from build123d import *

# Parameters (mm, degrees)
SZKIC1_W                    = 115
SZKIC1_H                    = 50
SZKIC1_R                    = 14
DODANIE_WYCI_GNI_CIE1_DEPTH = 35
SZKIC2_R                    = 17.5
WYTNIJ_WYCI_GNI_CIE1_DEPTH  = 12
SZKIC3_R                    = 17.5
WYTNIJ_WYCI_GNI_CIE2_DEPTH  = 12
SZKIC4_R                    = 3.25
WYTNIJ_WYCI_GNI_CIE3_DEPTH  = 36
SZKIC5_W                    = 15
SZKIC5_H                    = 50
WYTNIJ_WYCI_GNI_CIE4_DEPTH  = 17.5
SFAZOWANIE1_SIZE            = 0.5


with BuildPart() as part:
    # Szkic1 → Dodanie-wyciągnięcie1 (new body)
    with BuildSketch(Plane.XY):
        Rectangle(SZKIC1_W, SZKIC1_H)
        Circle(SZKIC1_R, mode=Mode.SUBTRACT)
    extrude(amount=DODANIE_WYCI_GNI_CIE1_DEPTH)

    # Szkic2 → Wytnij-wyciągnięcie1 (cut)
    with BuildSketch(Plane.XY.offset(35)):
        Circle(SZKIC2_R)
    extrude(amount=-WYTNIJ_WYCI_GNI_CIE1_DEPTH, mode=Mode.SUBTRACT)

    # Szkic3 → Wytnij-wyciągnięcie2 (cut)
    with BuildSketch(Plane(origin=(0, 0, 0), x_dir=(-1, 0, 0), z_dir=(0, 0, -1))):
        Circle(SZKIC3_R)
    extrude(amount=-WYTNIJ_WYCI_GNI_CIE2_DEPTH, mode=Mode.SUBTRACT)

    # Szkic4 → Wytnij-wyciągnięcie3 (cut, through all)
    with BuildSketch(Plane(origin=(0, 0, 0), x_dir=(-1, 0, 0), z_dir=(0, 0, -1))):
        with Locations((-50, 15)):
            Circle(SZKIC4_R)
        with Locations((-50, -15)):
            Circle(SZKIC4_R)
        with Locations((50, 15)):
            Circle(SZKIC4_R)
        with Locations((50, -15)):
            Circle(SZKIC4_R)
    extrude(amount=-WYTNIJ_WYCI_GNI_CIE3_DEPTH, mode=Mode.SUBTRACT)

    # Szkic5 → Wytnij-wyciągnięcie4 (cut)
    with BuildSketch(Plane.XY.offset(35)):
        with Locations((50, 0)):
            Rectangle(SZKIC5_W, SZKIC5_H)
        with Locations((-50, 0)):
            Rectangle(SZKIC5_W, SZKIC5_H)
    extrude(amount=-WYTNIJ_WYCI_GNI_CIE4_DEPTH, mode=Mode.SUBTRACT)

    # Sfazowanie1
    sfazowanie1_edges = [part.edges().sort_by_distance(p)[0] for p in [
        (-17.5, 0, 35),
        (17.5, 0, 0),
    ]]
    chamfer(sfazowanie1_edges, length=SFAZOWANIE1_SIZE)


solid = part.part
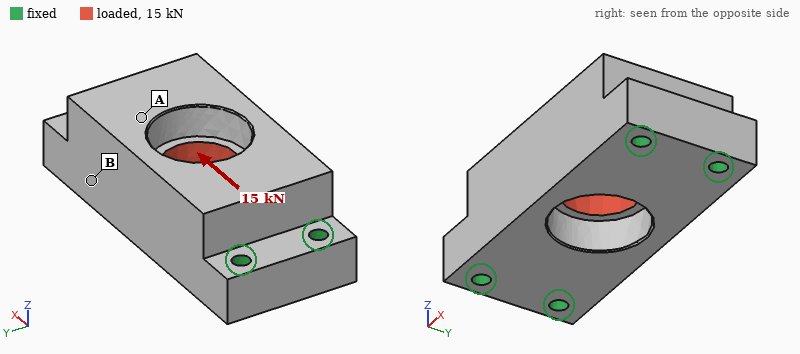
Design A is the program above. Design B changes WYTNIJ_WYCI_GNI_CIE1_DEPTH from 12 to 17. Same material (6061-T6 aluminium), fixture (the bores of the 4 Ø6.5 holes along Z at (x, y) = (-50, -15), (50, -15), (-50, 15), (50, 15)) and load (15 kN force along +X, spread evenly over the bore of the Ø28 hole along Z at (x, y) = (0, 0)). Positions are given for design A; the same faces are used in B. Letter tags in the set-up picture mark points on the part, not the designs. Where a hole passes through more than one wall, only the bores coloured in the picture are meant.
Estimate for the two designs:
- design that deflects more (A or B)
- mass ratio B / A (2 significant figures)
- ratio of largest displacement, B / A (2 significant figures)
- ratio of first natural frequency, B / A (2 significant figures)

B
0.99
1.2
1.0
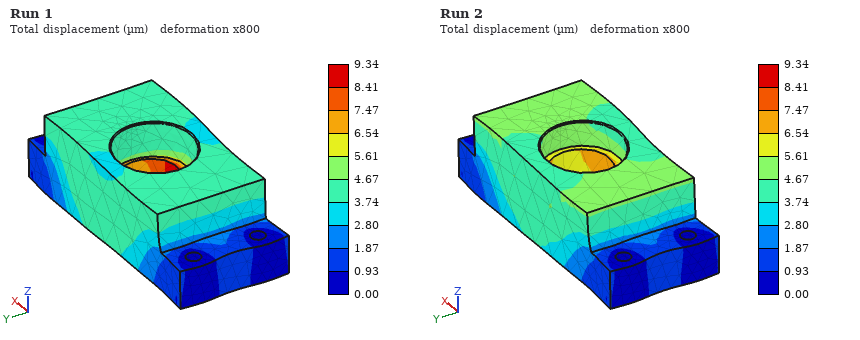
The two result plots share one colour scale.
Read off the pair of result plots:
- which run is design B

Run 1
